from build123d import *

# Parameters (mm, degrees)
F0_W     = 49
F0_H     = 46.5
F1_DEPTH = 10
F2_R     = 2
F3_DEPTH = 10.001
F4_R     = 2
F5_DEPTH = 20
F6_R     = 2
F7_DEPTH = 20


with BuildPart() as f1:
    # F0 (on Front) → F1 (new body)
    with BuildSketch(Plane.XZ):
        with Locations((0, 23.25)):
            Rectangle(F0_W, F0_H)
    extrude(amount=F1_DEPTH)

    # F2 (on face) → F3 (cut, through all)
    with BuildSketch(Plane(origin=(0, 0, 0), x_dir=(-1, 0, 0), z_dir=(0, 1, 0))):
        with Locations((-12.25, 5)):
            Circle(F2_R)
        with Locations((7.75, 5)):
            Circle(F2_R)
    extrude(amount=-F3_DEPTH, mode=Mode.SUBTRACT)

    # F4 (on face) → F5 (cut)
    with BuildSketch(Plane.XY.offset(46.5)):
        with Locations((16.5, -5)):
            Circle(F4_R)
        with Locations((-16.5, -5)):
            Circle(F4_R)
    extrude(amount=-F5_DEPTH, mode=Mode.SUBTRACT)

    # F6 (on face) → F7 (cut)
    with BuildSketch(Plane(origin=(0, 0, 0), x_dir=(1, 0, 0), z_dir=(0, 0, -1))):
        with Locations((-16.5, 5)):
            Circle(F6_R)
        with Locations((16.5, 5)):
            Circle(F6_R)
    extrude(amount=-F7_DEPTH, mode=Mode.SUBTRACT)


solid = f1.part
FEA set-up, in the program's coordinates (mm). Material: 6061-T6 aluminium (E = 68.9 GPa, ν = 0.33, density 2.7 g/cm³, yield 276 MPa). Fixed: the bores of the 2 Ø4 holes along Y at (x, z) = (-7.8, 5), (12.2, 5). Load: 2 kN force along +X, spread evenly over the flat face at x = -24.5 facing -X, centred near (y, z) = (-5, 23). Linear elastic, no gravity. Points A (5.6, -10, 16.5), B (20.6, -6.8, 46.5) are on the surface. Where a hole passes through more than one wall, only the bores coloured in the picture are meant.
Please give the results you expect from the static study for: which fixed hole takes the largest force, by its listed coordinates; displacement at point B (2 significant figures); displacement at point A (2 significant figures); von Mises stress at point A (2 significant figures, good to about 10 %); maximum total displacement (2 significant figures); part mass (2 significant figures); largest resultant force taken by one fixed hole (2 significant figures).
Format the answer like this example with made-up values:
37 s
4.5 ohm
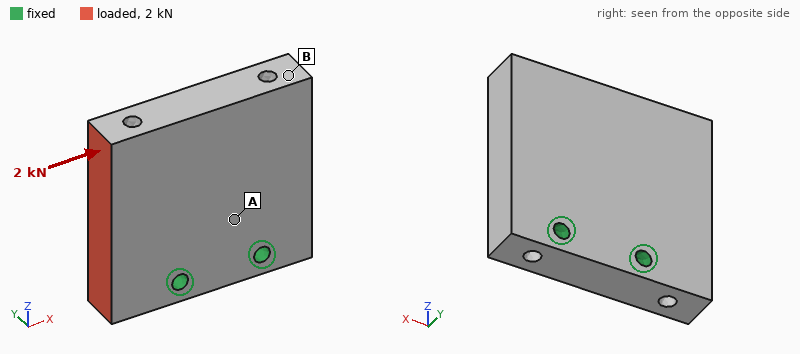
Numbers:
(-7.8, 5)
14 µm
3.7 µm
11 MPa
17 µm
58 g
2.0 kN
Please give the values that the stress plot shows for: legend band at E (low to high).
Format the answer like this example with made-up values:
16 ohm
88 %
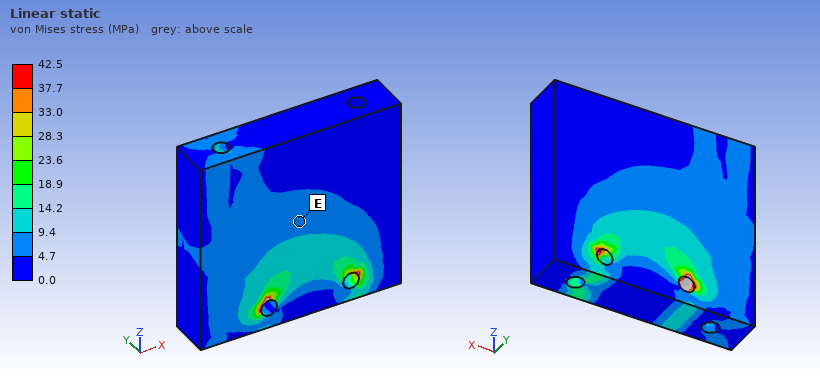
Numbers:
4.7 to 9.4 MPa
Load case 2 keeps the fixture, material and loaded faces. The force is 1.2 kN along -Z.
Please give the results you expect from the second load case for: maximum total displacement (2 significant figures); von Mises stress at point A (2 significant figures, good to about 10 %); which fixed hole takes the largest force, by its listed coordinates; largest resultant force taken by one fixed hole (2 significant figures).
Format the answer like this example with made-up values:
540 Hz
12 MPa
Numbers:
15 µm
5.6 MPa
(-7.8, 5)
2.0 kN
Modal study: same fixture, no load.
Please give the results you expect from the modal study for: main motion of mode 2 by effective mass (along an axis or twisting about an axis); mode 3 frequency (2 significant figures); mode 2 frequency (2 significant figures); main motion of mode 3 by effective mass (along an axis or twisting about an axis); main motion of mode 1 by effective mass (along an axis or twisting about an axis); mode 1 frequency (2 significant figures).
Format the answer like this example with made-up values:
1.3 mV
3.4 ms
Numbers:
twisting about Z
8700 Hz
7800 Hz
along X
along Y
4100 Hz
